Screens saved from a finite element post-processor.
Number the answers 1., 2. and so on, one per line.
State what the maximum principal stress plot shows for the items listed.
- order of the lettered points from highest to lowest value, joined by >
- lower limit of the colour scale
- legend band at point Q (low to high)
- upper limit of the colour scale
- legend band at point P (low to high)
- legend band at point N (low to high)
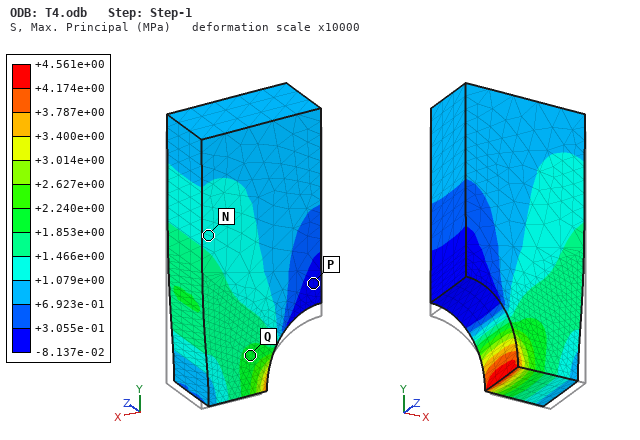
1. Q > N > P
2. -8.137e-02 MPa
3. +1.853e+00 to +2.240e+00 MPa
4. +4.561e+00 MPa
5. -8.137e-02 to +3.055e-01 MPa
6. +1.079e+00 to +1.466e+00 MPa
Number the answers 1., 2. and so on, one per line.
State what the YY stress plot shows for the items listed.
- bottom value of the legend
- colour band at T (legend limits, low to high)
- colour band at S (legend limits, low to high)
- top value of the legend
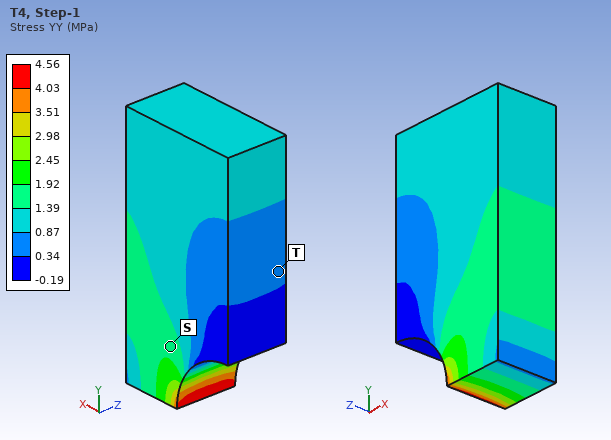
1. -0.19 MPa
2. 0.34 to 0.87 MPa
3. 1.39 to 1.92 MPa
4. 4.56 MPa
